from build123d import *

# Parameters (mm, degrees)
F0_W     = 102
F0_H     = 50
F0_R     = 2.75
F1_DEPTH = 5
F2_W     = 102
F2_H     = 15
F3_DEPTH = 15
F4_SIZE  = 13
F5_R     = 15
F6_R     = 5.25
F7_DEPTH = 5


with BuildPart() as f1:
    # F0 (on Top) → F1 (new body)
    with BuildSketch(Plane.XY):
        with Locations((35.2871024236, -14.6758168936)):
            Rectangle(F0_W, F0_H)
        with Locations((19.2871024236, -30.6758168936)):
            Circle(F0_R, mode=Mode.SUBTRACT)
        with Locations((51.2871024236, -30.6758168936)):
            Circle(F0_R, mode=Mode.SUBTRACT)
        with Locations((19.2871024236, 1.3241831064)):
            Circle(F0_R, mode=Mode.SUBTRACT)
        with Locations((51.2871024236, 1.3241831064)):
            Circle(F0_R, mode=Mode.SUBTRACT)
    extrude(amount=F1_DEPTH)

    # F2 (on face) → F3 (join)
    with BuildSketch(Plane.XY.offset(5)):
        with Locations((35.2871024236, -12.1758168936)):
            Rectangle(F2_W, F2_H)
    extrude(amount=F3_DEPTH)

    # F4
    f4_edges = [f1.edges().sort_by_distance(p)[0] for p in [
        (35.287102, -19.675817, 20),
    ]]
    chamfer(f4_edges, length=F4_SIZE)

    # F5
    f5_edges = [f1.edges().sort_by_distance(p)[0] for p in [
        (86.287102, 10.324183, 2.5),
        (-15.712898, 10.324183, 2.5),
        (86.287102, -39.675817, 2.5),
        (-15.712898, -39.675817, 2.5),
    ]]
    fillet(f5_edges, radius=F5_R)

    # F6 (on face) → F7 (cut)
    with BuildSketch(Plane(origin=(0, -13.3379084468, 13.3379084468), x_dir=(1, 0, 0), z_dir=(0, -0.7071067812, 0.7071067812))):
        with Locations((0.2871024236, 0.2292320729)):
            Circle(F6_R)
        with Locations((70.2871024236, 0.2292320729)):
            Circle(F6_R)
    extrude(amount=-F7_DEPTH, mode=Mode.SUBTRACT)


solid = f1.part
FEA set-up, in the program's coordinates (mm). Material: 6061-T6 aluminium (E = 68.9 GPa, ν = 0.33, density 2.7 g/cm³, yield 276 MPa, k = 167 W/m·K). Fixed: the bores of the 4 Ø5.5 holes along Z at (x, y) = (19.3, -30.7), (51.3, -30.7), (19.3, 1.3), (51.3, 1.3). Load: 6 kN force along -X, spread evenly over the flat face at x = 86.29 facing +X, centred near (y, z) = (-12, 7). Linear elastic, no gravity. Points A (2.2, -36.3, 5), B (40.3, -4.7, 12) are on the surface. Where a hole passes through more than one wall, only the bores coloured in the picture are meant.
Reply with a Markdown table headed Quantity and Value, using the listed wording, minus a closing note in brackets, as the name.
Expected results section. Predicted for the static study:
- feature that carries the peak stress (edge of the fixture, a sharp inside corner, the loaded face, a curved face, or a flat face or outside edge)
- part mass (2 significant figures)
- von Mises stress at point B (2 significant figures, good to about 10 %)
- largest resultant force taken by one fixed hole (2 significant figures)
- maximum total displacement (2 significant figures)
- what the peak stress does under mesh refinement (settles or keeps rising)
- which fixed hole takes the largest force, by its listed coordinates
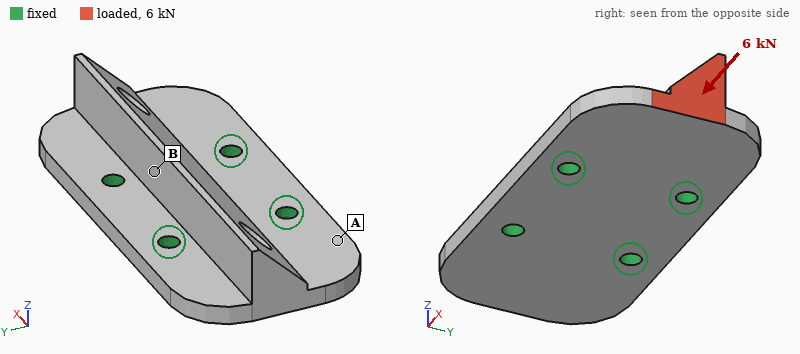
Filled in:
| Quantity | Value |
|---|---|
| feature that carries the peak stress | edge of the fixture |
| part mass | 100 g |
| von Mises stress at point B | 16 MPa |
| largest resultant force taken by one fixed hole | 2.4 kN |
| maximum total displacement | 54 µm |
| what the peak stress does under mesh refinement | keeps rising |
| which fixed hole takes the largest force, by its listed coordinates | (51.3, 1.3) |
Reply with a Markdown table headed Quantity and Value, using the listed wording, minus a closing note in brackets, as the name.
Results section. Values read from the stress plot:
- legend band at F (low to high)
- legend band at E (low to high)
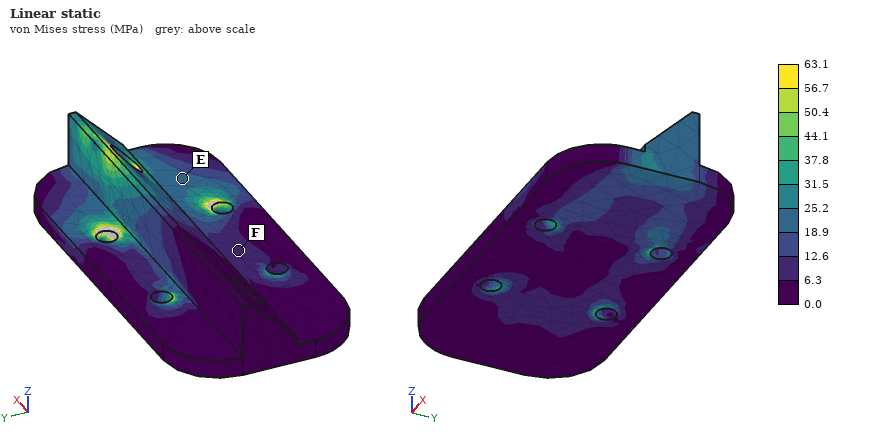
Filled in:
| Quantity | Value |
|---|---|
| legend band at F | 6.3 to 12.6 MPa |
| legend band at E | 18.9 to 25.2 MPa |
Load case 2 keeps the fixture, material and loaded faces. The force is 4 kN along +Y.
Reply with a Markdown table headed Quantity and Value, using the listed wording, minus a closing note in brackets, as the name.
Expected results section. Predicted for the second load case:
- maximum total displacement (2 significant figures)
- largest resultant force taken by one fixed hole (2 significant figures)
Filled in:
| Quantity | Value |
|---|---|
| maximum total displacement | 94 µm |
| largest resultant force taken by one fixed hole | 4.2 kN |
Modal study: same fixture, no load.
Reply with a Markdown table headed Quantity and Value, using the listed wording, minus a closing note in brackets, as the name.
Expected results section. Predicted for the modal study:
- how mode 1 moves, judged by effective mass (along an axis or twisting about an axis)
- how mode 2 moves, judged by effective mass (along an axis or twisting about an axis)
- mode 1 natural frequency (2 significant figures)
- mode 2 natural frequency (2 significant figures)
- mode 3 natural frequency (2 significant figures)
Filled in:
| Quantity | Value |
|---|---|
| how mode 1 moves, judged by effective mass | twisting about Y |
| how mode 2 moves, judged by effective mass | along Z |
| mode 1 natural frequency | 5200 Hz |
| mode 2 natural frequency | 6200 Hz |
| mode 3 natural frequency | 9300 Hz |
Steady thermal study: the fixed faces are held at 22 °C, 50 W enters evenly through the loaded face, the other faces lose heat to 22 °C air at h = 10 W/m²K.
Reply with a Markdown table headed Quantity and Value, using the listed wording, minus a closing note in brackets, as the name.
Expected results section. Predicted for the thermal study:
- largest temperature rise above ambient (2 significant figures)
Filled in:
| Quantity | Value |
|---|---|
| largest temperature rise above ambient | 40 K |
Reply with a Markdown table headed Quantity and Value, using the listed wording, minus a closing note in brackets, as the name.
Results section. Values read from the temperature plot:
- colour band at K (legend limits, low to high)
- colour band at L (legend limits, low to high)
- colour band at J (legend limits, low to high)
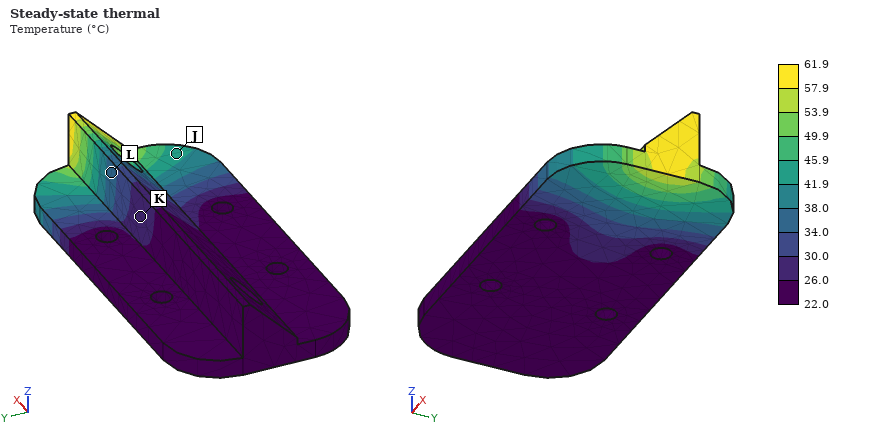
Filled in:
| Quantity | Value |
|---|---|
| colour band at K | 26.0 to 30.0 °C |
| colour band at L | 34.0 to 38.0 °C |
| colour band at J | 41.9 to 45.9 °C |
